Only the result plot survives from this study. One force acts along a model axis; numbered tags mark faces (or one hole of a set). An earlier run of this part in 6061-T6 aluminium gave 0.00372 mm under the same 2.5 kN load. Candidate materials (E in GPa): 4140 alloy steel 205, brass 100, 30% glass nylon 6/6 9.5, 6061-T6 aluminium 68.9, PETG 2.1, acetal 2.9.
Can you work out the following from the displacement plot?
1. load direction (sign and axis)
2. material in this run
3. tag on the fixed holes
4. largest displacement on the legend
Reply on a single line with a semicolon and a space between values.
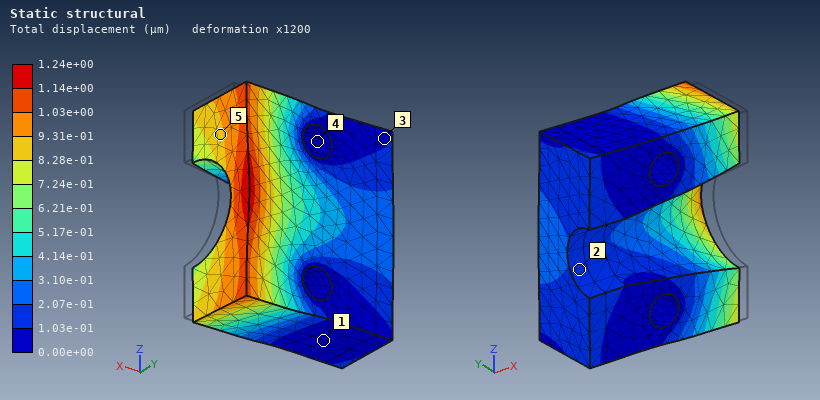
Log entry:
-X; 4140 alloy steel; 4; 1.24e+00 µm
